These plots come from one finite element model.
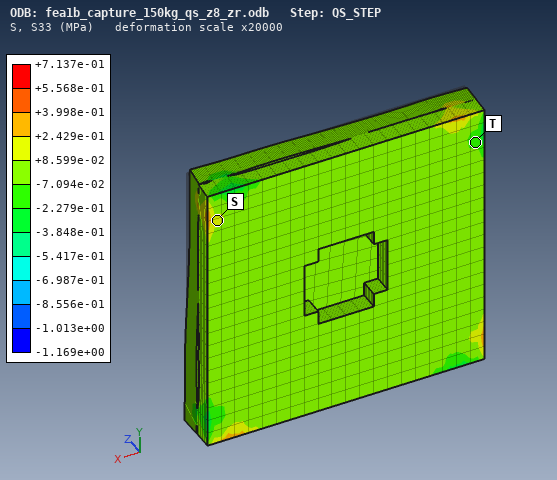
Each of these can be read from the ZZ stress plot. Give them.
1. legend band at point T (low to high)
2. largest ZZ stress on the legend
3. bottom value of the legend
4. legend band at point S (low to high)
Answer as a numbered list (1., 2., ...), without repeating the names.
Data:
1. -2.279e-01 to -7.094e-02 MPa
2. +7.137e-01 MPa
3. -1.169e+00 MPa
4. +8.599e-02 to +2.429e-01 MPa
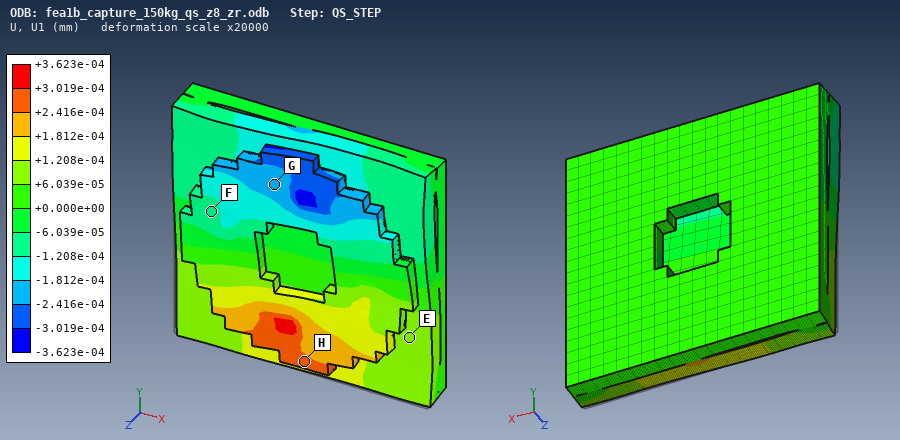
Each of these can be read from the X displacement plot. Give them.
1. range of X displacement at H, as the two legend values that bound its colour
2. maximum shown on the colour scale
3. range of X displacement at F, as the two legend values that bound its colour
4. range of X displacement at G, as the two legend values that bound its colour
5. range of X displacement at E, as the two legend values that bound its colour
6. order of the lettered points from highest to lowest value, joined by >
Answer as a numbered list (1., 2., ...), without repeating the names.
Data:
1. +2.416e-04 to +3.019e-04 mm
2. +3.623e-04 mm
3. -1.208e-04 to -6.039e-05 mm
4. -2.416e-04 to -1.812e-04 mm
5. +6.039e-05 to +1.208e-04 mm
6. H > E > F > G
